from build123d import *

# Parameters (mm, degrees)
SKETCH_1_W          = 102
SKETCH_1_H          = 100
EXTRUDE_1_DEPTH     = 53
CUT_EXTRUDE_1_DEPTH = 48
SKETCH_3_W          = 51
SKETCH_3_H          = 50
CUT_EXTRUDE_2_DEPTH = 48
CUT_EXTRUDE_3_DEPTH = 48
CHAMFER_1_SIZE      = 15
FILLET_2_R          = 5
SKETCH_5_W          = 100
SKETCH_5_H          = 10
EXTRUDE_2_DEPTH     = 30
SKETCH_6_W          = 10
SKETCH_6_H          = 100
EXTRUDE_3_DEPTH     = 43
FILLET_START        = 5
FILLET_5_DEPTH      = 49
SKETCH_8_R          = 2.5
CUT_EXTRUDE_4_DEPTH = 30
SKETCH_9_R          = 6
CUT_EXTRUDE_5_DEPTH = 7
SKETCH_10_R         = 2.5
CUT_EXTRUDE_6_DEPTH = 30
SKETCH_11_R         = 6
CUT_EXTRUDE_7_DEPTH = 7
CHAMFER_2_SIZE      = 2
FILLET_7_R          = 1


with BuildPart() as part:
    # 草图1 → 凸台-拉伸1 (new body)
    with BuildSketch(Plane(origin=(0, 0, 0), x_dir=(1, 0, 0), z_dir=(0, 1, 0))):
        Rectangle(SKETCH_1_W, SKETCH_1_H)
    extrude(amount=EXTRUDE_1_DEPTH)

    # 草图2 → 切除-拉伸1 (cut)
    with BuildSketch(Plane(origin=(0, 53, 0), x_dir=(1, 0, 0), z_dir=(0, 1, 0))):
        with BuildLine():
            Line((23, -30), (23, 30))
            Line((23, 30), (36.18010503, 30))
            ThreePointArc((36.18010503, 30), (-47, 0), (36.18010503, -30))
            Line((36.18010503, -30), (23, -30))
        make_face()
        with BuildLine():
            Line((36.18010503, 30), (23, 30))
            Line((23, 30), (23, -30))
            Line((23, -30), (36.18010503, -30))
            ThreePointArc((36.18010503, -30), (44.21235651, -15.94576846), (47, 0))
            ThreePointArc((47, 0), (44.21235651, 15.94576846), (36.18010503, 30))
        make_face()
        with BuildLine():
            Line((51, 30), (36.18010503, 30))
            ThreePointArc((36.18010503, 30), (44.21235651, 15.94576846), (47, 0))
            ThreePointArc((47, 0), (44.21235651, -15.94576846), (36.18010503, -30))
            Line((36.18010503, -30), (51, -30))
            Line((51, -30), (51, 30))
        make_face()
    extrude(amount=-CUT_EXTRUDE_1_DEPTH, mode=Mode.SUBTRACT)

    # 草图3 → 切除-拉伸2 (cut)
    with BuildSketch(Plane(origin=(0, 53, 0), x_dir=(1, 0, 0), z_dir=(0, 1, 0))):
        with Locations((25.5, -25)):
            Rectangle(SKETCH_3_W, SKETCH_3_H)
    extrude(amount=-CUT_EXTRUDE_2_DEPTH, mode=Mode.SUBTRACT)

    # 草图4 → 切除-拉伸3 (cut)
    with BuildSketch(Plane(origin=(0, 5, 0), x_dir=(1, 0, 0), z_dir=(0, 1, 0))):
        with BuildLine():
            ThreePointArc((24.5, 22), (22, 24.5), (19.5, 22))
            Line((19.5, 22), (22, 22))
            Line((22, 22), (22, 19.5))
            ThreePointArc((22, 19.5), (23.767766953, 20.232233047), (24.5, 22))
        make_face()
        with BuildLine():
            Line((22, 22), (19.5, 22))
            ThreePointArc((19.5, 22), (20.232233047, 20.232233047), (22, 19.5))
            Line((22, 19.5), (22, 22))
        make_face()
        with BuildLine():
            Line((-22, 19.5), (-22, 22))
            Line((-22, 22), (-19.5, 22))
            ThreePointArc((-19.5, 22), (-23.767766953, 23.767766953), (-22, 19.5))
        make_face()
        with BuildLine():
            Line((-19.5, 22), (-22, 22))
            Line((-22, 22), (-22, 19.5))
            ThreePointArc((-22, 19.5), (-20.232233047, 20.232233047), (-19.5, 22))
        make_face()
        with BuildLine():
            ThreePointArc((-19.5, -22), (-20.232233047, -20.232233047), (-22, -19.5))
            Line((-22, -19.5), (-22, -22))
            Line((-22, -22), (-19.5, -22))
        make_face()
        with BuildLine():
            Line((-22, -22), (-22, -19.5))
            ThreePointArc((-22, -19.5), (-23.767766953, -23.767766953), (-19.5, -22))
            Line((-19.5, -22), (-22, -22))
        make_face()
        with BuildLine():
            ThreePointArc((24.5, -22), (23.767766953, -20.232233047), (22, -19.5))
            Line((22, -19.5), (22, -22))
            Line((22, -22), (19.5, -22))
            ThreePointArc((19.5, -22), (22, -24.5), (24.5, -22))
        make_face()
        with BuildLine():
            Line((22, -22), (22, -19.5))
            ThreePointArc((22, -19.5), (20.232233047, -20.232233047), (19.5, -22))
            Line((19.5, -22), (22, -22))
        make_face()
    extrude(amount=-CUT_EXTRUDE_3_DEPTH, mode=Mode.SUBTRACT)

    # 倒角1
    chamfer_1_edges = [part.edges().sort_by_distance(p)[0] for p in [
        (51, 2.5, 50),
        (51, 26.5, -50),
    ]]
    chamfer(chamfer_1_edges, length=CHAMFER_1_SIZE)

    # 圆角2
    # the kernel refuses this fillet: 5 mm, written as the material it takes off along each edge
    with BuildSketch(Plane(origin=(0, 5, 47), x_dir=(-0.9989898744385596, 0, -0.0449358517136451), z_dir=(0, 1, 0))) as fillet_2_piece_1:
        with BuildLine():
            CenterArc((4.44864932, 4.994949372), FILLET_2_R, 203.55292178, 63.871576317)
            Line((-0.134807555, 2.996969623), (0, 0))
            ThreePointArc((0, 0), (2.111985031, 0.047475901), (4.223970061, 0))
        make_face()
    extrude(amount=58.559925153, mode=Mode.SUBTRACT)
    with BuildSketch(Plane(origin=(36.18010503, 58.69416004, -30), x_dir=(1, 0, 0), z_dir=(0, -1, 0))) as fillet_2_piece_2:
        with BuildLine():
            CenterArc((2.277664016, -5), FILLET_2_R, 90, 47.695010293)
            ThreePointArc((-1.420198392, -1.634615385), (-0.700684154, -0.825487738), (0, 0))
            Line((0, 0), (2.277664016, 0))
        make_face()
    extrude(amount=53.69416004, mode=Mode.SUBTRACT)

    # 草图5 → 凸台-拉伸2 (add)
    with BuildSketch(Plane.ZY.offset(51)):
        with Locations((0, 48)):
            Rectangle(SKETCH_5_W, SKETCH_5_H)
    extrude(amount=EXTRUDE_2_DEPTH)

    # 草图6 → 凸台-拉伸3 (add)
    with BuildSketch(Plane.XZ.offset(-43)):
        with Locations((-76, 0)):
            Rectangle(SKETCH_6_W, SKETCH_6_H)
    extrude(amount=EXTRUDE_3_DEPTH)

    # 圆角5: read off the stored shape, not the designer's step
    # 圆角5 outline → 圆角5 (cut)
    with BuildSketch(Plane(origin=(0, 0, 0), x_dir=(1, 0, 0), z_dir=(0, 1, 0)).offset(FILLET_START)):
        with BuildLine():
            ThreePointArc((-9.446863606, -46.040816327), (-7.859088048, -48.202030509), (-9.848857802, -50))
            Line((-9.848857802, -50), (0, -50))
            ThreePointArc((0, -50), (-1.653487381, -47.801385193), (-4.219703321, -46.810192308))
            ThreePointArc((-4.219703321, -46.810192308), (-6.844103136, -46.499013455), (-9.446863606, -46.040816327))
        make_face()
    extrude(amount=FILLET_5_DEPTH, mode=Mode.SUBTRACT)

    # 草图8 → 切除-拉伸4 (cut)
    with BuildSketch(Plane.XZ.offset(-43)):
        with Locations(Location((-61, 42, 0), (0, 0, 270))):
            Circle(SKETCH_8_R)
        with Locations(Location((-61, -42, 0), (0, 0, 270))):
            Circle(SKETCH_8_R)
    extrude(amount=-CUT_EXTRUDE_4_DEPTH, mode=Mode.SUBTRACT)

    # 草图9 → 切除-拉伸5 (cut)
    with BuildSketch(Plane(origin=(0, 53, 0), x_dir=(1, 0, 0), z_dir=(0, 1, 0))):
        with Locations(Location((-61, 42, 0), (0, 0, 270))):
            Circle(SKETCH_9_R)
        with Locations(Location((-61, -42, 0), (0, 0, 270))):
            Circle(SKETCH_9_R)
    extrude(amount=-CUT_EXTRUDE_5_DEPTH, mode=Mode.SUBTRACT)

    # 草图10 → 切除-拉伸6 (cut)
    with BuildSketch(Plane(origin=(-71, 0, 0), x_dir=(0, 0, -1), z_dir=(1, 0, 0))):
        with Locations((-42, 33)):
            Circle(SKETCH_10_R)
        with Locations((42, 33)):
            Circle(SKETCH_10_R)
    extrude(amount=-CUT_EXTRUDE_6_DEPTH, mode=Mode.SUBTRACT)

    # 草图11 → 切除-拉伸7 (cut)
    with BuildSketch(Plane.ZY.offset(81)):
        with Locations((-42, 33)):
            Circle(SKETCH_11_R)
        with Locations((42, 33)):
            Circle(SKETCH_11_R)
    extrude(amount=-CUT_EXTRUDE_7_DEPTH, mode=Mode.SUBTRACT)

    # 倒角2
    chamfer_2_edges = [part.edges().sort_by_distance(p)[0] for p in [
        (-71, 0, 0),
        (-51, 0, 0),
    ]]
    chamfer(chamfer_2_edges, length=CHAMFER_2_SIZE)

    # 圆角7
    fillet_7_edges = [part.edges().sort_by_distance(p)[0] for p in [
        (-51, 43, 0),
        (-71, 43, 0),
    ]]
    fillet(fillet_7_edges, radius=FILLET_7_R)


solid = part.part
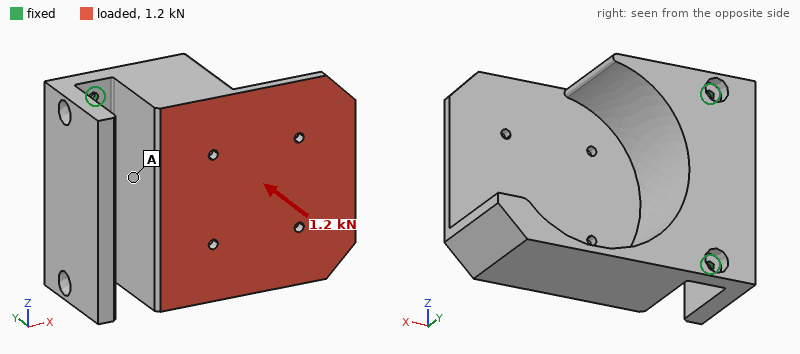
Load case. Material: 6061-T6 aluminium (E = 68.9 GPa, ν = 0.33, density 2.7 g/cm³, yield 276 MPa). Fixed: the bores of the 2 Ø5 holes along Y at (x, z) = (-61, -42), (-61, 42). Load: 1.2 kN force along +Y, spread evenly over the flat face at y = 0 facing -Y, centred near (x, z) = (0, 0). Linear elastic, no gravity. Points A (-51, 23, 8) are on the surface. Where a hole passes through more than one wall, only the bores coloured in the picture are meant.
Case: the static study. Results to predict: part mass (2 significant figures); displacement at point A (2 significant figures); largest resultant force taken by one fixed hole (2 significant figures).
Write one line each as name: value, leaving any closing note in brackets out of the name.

part mass: 590 g
displacement at point A: 0.35 mm
largest resultant force taken by one fixed hole: 650 N
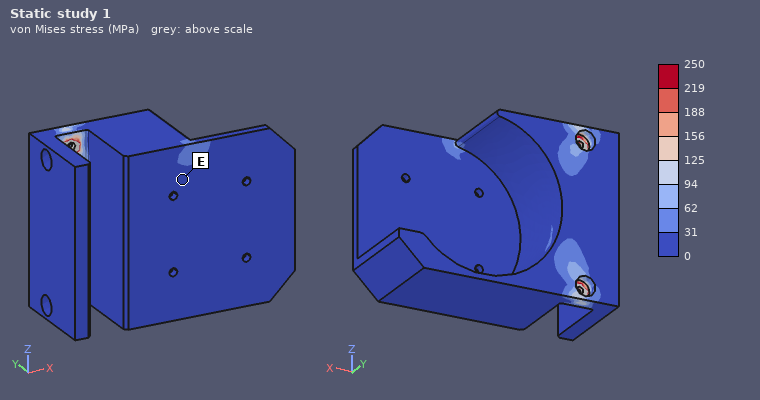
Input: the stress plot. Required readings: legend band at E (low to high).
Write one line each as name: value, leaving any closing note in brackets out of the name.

legend band at E: 0 to 31 MPa
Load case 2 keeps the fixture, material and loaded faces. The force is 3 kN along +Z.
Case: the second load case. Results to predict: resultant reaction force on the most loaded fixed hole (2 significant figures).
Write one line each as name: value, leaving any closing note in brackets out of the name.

resultant reaction force on the most loaded fixed hole: 3.1 kN
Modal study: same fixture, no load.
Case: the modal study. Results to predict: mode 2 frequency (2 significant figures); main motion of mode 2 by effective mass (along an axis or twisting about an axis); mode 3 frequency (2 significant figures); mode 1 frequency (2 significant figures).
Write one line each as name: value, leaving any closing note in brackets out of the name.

mode 2 frequency: 1000 Hz
main motion of mode 2 by effective mass: along Z
mode 3 frequency: 1500 Hz
mode 1 frequency: 270 Hz
